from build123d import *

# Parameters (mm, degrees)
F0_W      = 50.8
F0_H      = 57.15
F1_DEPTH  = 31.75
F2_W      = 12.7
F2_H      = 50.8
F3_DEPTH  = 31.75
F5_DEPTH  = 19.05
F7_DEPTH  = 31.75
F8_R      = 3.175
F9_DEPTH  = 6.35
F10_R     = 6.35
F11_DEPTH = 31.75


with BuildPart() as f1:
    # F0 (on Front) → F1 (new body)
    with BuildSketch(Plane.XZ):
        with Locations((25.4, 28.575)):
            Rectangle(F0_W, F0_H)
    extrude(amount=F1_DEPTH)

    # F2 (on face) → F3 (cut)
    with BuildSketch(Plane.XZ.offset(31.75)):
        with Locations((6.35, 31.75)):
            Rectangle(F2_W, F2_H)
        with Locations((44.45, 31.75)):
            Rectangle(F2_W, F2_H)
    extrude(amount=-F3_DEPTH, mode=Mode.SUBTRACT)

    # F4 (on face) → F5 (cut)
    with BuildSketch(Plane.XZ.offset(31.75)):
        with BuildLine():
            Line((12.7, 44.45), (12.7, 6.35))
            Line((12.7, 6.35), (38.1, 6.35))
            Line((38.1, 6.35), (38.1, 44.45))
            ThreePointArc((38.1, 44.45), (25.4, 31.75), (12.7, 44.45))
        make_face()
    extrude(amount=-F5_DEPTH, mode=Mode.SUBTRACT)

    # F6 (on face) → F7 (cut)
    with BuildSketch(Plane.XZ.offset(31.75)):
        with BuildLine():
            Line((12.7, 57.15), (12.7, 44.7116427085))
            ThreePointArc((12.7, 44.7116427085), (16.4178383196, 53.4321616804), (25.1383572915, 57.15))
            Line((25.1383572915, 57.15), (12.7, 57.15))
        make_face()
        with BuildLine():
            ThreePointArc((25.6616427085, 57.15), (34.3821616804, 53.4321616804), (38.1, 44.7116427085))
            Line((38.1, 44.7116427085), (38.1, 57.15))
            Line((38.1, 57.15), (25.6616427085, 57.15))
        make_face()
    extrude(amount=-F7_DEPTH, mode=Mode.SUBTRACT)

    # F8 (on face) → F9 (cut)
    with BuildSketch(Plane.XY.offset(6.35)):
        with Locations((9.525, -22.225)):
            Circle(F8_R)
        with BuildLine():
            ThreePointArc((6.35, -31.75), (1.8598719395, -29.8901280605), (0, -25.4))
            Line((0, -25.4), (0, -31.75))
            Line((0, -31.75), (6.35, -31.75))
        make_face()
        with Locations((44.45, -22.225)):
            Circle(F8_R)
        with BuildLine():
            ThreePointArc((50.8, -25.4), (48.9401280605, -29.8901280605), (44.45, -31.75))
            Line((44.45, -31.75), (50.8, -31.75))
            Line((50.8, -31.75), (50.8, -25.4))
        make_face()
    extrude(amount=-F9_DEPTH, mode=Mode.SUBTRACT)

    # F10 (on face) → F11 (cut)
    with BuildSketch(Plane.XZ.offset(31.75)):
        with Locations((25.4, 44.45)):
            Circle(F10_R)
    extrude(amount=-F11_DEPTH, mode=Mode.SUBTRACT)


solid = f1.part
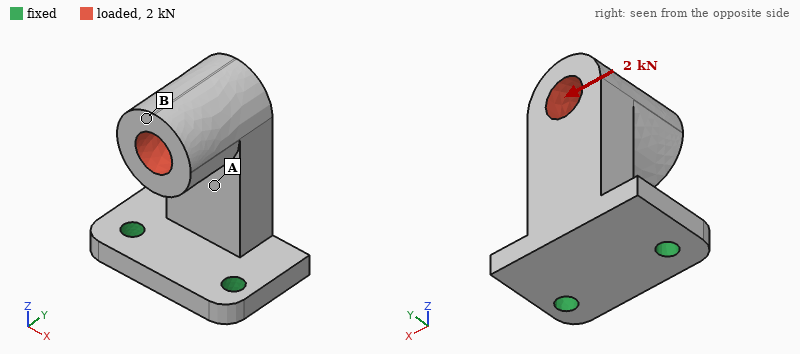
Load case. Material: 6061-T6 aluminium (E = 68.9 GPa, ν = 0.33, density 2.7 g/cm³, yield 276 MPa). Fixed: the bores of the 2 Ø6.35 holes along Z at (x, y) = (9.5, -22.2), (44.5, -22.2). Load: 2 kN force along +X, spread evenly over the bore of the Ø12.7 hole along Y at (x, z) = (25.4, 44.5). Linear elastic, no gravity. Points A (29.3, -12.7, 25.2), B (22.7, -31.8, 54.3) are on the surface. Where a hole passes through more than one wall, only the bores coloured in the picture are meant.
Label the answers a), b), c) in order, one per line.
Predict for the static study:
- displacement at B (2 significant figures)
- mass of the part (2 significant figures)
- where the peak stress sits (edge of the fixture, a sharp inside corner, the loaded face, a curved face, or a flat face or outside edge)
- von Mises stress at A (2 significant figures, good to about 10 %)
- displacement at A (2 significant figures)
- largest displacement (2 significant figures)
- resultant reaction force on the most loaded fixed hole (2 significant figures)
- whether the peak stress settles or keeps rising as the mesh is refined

a) 0.29 mm
b) 83 g
c) edge of the fixture
d) 49 MPa
e) 0.099 mm
f) 0.30 mm
g) 2.8 kN
h) keeps rising
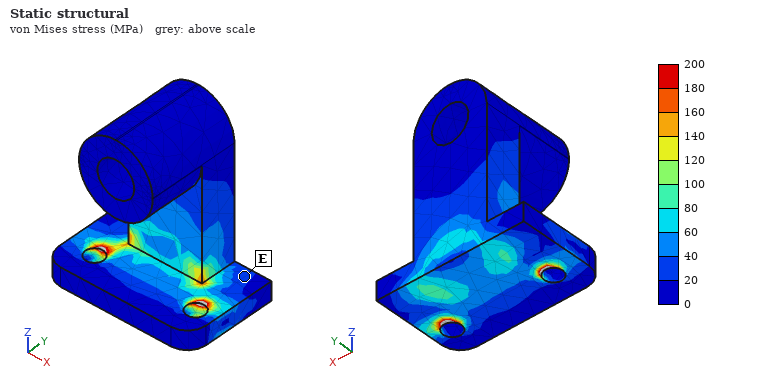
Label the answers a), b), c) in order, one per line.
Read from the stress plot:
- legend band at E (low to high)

a) 20 to 40 MPa
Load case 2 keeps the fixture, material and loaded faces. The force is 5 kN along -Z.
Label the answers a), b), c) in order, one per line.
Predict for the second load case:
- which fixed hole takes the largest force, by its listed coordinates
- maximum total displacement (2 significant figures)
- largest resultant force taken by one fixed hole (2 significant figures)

a) (9.5, -22.2)
b) 0.27 mm
c) 2.7 kN
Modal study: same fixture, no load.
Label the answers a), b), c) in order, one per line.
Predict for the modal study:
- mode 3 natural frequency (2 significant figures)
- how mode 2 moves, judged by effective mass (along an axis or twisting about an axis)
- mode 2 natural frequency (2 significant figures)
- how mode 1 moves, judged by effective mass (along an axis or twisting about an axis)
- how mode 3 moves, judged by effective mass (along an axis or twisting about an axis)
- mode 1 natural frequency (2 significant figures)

a) 5200 Hz
b) along X
c) 2500 Hz
d) along Y
e) along Z
f) 1300 Hz
